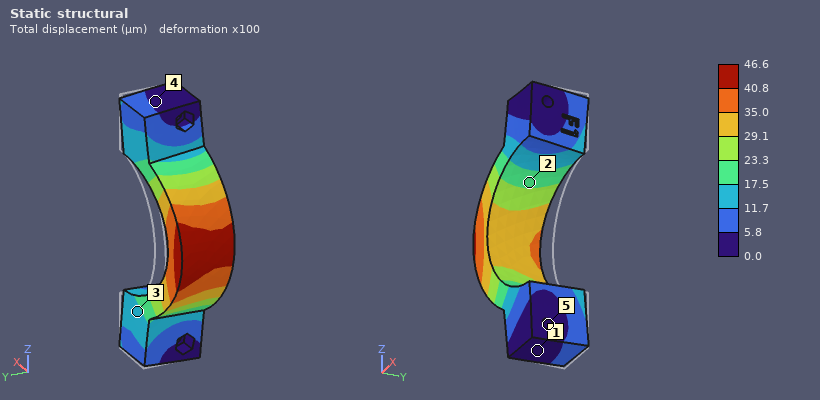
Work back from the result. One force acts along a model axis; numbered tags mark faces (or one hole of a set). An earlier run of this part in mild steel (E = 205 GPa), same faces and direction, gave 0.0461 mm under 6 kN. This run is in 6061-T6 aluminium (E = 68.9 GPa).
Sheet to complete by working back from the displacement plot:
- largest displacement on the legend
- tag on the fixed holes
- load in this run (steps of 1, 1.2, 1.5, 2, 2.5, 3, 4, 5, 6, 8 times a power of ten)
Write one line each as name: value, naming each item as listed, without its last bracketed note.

largest displacement on the legend: 46.6 µm
tag on the fixed holes: 5
load in this run: 2 kN
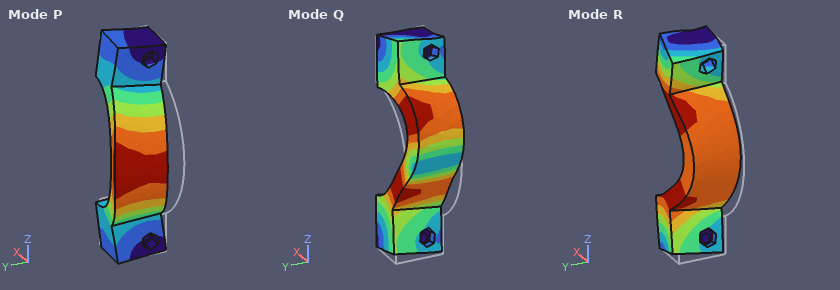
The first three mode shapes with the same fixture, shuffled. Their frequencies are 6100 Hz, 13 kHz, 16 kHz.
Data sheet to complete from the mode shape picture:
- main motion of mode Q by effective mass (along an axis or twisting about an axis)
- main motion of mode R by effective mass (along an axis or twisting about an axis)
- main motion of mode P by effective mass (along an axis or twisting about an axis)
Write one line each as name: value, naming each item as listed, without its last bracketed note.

main motion of mode Q by effective mass: along Z
main motion of mode R by effective mass: along X
main motion of mode P by effective mass: along Y
